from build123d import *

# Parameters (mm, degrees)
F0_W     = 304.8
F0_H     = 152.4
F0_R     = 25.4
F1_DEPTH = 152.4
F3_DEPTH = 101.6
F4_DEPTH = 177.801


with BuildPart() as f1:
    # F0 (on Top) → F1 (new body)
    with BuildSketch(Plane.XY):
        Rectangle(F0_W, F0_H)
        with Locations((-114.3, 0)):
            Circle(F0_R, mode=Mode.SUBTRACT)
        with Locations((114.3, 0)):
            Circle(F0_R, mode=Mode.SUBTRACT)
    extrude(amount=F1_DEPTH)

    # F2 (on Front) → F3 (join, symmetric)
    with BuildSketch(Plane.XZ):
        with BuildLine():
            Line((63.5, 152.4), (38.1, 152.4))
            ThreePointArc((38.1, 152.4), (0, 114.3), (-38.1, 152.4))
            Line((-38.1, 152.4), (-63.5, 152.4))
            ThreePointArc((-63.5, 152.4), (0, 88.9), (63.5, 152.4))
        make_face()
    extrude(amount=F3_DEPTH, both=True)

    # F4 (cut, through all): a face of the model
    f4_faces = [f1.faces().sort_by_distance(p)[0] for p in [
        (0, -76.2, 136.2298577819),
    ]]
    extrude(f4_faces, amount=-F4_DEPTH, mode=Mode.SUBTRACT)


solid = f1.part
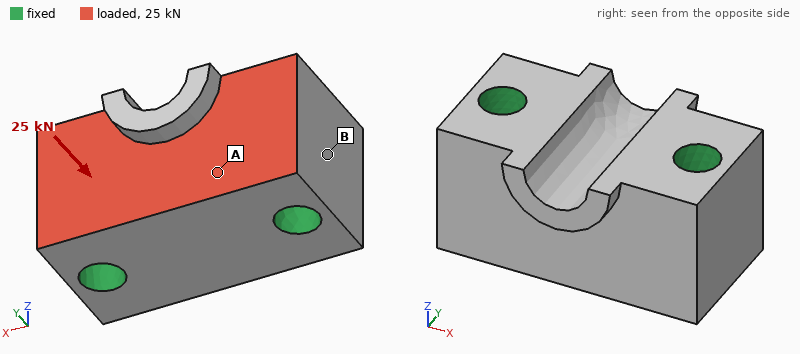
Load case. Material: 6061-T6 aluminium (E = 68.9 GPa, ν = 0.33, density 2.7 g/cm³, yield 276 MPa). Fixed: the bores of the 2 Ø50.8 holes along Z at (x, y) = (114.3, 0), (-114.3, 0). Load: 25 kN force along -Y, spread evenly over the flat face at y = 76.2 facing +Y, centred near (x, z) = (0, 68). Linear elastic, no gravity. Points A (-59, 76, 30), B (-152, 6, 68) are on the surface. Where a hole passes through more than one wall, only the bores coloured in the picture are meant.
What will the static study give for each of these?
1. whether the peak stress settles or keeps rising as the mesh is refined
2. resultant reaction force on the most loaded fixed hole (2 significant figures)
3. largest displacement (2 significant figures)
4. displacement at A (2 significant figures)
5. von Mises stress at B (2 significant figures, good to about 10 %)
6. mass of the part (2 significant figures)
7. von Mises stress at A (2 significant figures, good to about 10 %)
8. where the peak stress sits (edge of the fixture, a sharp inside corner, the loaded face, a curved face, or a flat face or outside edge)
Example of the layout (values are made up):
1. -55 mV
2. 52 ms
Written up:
1. keeps rising
2. 13 kN
3. 1.9 µm
4. 1.2 µm
5. 0.29 MPa
6. 17 kg
7. 0.56 MPa
8. edge of the fixture
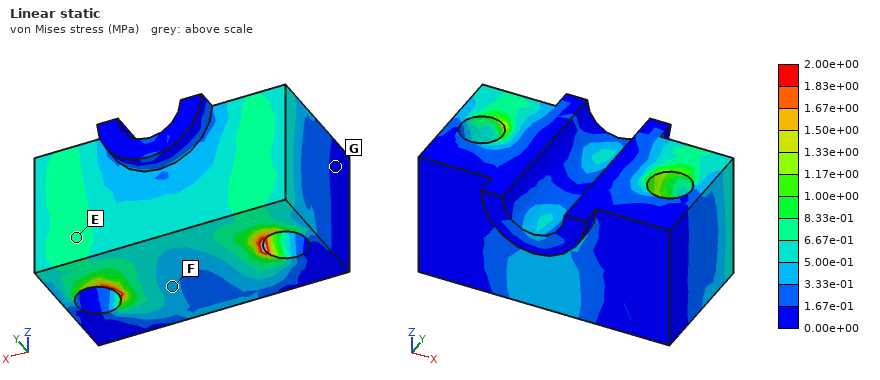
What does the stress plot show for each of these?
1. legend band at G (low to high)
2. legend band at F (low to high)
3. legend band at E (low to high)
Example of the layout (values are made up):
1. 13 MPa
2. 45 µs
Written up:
1. 0.00e+00 to 1.67e-01 MPa
2. 3.33e-01 to 5.00e-01 MPa
3. 6.67e-01 to 8.33e-01 MPa
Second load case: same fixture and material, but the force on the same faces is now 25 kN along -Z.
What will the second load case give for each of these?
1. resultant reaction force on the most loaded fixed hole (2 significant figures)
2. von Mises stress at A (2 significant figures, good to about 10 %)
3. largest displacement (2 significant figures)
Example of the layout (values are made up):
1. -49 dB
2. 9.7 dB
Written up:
1. 13 kN
2. 1.5 MPa
3. 4.6 µm
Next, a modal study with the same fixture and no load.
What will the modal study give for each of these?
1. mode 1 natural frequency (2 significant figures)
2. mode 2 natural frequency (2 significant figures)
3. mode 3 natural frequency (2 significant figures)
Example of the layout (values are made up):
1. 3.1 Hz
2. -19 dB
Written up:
1. 5800 Hz
2. 6000 Hz
3. 6500 Hz
